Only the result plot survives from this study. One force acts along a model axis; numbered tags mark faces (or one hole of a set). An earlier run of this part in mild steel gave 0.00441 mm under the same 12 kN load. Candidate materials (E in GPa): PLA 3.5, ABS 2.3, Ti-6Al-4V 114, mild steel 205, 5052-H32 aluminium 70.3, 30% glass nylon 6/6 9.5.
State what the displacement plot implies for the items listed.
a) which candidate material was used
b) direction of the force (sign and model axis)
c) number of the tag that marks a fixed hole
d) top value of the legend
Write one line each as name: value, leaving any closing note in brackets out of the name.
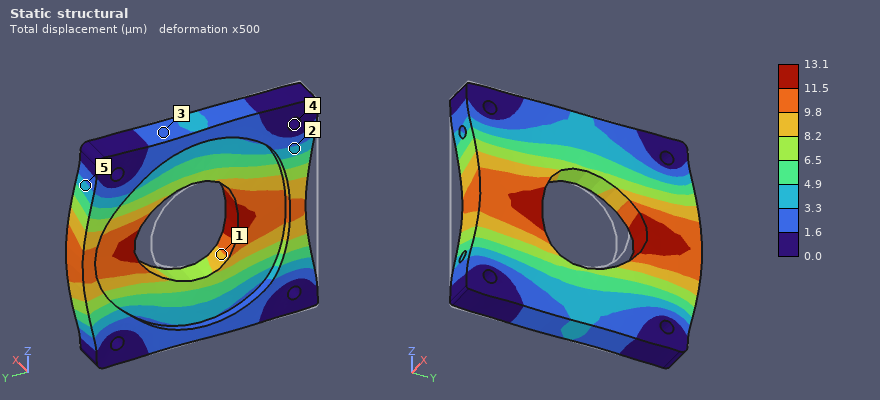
which candidate material was used: 5052-H32 aluminium
direction of the force: +Y
number of the tag that marks a fixed hole: 4
top value of the legend: 13.1 µm
